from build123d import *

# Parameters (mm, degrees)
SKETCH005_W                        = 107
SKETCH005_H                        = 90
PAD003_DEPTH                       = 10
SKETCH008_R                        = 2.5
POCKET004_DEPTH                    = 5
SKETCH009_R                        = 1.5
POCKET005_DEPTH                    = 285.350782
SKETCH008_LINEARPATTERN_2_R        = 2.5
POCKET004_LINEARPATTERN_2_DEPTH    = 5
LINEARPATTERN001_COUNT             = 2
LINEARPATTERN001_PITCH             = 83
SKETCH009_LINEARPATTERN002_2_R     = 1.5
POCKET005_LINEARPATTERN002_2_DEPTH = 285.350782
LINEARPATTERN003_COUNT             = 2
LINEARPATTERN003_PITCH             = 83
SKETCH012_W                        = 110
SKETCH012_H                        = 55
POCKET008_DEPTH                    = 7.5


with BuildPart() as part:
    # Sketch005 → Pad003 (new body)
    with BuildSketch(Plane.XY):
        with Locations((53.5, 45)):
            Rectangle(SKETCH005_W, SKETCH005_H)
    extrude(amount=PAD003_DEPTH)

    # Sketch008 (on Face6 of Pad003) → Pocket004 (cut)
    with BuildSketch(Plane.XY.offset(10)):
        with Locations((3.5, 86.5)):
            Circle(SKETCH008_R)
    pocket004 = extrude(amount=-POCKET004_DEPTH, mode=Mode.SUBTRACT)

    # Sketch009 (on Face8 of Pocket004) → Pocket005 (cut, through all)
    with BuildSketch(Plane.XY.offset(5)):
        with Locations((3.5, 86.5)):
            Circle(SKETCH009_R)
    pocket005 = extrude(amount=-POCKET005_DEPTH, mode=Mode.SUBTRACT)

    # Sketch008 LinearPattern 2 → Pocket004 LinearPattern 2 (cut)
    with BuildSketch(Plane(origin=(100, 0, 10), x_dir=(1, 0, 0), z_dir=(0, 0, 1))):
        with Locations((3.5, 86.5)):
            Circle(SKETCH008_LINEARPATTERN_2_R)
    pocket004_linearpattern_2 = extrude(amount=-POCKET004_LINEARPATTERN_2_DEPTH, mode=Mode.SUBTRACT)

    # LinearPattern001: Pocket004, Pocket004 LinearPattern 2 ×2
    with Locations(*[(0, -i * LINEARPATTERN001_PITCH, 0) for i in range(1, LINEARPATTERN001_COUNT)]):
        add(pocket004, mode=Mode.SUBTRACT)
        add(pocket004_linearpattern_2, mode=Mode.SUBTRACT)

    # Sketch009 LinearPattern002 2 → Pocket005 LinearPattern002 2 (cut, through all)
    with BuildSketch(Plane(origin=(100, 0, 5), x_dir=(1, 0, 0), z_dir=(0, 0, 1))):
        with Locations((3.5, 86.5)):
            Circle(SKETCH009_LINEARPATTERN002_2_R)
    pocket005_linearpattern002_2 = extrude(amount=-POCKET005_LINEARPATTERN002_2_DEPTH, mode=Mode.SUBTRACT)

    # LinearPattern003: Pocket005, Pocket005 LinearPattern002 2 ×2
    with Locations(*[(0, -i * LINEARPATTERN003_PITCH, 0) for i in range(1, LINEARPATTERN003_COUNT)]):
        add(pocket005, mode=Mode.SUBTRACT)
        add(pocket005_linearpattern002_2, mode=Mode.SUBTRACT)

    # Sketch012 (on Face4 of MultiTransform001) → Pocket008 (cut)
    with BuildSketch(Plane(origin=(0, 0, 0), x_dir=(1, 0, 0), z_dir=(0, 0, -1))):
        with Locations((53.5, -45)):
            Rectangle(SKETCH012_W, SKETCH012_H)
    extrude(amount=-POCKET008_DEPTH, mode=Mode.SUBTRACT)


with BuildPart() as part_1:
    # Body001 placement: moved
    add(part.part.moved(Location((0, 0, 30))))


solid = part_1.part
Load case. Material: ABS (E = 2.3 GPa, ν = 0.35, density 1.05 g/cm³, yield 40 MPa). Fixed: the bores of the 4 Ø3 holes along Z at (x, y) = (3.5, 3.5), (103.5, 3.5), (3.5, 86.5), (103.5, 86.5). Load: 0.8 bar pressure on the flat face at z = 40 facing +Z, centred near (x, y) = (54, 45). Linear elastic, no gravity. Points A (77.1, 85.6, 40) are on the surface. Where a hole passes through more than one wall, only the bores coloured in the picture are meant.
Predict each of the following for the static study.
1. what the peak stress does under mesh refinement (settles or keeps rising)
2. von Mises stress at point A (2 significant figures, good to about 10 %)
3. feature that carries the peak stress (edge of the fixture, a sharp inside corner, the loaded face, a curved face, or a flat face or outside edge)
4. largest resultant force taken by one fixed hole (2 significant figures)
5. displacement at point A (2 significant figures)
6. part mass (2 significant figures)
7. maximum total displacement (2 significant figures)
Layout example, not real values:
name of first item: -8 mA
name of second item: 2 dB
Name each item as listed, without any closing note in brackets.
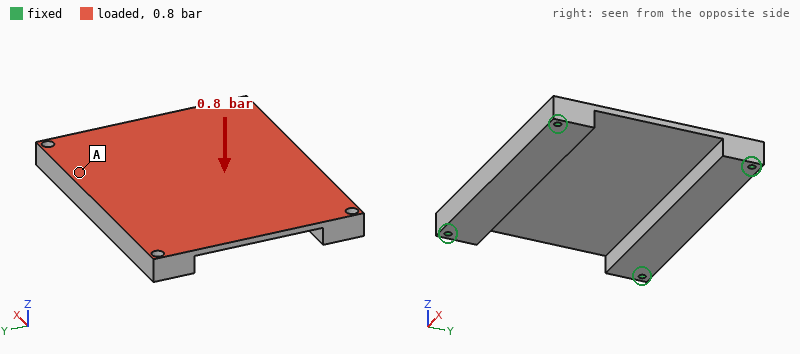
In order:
what the peak stress does under mesh refinement: keeps rising
von Mises stress at point A: 3.5 MPa
feature that carries the peak stress: edge of the fixture
largest resultant force taken by one fixed hole: 490 N
displacement at point A: 0.30 mm
part mass: 54 g
maximum total displacement: 1.5 mm
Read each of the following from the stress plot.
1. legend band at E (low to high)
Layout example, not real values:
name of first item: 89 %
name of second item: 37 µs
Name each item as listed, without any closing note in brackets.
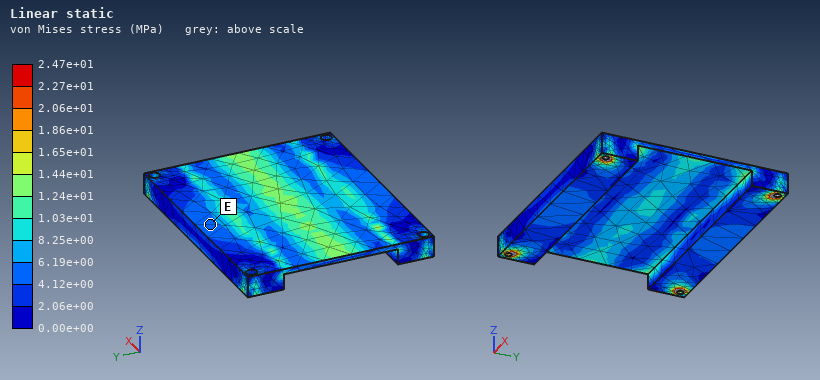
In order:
legend band at E: 4.12e+00 to 6.19e+00 MPa
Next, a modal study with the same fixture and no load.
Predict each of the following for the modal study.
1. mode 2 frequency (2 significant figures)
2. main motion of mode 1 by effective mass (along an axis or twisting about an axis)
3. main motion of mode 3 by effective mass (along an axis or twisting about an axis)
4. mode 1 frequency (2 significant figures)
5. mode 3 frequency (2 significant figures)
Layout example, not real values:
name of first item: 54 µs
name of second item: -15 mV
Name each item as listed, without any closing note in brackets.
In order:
mode 2 frequency: 940 Hz
main motion of mode 1 by effective mass: along Z
main motion of mode 3 by effective mass: twisting about Y
mode 1 frequency: 820 Hz
mode 3 frequency: 1200 Hz
